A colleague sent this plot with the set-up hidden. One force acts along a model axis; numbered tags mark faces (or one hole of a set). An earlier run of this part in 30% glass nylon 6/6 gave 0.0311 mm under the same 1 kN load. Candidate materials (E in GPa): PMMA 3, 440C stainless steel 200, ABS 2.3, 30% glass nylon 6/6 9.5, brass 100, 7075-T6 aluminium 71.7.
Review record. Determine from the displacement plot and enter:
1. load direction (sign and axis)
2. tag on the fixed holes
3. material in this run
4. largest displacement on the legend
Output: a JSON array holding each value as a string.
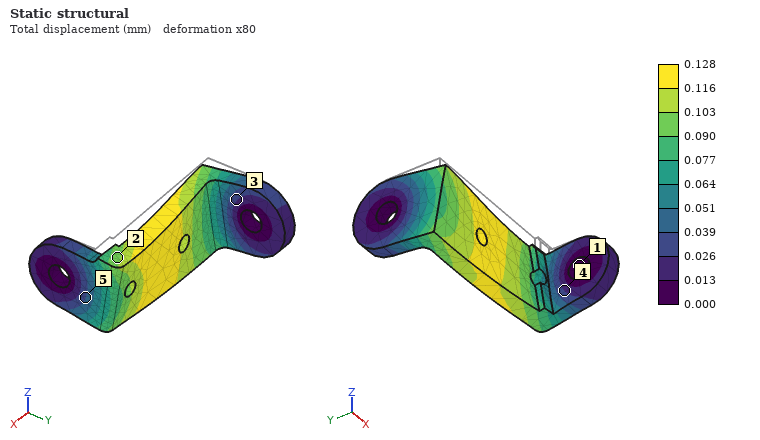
["-Z", "1", "ABS", "0.128 mm"]
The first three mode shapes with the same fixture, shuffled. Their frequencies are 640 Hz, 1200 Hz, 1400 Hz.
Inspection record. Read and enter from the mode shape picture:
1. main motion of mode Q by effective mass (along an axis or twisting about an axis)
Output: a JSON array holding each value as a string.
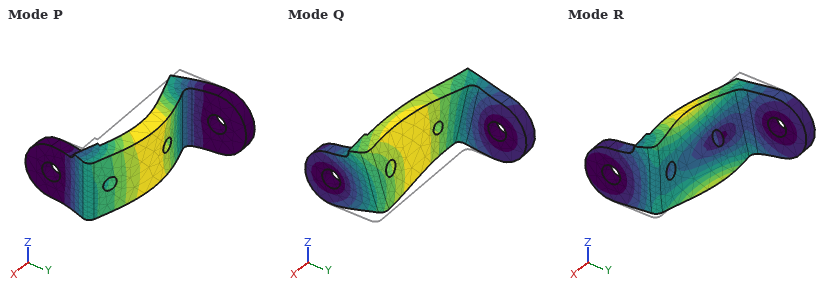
["along Z"]
